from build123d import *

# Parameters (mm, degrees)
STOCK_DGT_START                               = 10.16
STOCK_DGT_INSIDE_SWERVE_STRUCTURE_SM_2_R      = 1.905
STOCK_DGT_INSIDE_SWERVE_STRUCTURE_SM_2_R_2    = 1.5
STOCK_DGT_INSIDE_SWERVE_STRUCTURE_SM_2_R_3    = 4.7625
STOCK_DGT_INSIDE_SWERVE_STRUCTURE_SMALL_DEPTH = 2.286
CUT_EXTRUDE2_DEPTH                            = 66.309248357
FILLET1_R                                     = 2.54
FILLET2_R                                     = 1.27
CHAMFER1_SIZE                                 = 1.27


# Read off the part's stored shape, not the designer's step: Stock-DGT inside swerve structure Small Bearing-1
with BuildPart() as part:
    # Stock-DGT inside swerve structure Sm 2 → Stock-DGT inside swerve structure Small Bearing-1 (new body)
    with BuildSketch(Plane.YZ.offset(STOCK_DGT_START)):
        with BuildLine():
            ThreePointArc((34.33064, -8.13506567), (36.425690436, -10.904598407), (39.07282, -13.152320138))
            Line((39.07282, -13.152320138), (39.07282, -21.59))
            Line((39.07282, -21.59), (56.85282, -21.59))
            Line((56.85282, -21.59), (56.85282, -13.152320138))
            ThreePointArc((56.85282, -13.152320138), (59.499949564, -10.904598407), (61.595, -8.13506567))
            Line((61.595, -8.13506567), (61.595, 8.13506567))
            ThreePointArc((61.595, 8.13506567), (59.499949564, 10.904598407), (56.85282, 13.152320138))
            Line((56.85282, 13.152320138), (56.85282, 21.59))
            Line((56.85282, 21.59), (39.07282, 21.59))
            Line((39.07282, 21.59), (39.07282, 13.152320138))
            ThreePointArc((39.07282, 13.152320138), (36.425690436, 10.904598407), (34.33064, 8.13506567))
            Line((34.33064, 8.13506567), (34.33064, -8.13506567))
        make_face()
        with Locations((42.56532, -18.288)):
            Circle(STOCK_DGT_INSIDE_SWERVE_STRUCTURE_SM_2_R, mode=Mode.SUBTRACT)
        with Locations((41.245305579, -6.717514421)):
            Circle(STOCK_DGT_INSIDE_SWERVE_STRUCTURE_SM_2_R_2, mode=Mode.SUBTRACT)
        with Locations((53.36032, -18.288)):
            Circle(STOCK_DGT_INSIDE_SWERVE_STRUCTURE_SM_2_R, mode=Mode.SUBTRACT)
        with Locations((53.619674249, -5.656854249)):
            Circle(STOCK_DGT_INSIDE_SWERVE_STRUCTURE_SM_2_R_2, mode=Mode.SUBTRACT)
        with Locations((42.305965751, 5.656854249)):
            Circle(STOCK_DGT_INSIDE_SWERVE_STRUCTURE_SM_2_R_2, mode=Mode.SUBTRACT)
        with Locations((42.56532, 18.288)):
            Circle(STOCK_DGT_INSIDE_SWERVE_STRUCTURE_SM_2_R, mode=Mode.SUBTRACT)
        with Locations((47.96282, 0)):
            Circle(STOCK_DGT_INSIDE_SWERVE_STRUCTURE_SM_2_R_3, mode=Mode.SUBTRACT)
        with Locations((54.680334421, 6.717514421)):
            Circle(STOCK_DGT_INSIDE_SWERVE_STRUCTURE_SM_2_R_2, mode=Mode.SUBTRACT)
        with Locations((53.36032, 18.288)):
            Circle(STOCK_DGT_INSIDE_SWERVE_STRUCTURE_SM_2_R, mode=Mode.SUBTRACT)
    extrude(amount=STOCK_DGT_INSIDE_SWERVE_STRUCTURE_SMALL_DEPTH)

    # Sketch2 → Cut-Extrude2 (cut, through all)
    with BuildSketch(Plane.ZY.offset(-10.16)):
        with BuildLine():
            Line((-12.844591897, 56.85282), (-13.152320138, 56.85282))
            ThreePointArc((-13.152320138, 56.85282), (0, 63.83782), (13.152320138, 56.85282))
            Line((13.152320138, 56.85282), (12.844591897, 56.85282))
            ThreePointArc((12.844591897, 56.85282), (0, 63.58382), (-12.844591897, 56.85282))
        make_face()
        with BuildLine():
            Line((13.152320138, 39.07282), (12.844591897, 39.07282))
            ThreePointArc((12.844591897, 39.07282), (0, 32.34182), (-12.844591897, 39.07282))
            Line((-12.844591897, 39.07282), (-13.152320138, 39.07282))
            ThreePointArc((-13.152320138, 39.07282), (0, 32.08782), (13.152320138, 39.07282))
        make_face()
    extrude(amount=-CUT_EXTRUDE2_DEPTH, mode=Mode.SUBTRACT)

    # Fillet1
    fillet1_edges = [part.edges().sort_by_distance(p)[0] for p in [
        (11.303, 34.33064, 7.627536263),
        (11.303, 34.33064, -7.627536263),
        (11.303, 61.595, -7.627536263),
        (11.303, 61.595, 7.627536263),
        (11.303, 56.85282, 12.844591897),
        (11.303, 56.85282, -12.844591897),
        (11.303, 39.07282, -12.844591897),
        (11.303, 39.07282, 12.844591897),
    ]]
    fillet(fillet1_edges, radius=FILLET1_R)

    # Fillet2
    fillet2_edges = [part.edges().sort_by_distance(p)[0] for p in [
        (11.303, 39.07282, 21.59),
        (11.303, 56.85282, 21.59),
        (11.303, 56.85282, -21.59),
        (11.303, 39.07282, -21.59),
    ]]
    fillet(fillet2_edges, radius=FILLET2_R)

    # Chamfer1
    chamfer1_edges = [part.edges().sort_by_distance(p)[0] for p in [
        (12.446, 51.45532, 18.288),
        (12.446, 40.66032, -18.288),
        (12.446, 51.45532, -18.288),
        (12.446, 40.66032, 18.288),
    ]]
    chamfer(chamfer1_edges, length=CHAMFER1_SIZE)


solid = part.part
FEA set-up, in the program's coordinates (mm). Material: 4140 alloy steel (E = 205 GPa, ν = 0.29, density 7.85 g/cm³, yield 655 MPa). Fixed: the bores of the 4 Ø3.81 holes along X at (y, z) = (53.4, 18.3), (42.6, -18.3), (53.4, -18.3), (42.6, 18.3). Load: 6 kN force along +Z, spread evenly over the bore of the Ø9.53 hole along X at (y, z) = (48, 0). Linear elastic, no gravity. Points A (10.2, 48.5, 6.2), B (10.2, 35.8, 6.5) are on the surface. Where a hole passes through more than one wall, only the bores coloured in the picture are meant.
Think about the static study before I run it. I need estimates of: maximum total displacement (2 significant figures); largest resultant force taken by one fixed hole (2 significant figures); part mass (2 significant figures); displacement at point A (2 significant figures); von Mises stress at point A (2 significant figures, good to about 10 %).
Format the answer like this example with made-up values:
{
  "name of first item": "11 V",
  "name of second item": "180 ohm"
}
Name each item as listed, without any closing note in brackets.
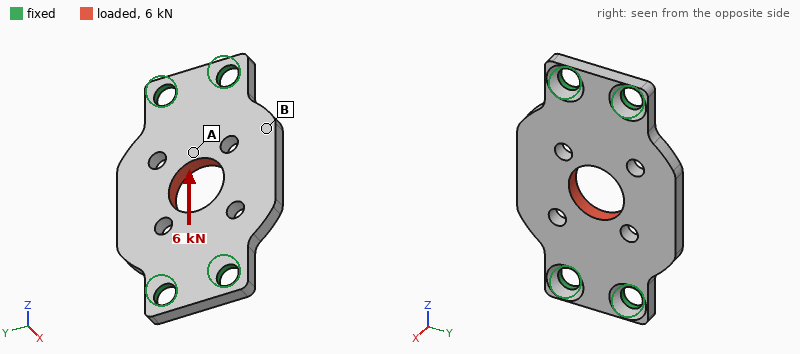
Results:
{
  "maximum total displacement": "9.4 µm",
  "largest resultant force taken by one fixed hole": "1.5 kN",
  "part mass": "14 g",
  "displacement at point A": "6.5 µm",
  "von Mises stress at point A": "89 MPa"
}
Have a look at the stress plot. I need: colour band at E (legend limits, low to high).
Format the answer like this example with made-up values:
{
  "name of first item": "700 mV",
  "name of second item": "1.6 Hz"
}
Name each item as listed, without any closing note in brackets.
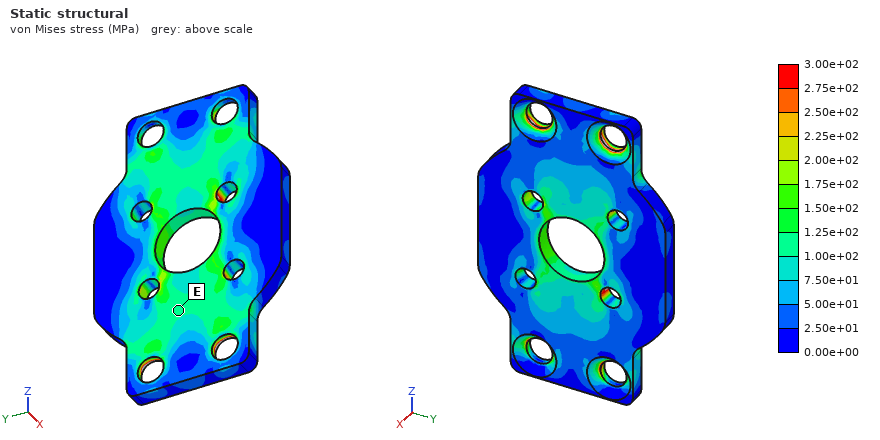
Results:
{
  "colour band at E": "1.00e+02 to 1.25e+02 MPa"
}
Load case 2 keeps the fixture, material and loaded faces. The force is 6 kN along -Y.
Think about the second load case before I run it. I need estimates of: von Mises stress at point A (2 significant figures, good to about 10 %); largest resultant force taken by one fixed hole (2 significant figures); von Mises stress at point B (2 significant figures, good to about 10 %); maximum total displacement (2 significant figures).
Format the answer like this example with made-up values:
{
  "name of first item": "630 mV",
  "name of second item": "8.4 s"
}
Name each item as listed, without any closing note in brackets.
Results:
{
  "von Mises stress at point A": "170 MPa",
  "largest resultant force taken by one fixed hole": "1.9 kN",
  "von Mises stress at point B": "80 MPa",
  "maximum total displacement": "19 µm"
}
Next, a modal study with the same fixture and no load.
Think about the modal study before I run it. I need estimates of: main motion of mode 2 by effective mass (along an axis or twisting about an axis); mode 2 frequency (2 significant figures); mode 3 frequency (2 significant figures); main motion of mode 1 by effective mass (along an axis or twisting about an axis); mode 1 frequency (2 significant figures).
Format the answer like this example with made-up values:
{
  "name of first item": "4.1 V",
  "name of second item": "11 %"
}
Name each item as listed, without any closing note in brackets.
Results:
{
  "main motion of mode 2 by effective mass": "twisting about Z",
  "mode 2 frequency": "8400 Hz",
  "mode 3 frequency": "19 kHz",
  "main motion of mode 1 by effective mass": "along X",
  "mode 1 frequency": "7300 Hz"
}
